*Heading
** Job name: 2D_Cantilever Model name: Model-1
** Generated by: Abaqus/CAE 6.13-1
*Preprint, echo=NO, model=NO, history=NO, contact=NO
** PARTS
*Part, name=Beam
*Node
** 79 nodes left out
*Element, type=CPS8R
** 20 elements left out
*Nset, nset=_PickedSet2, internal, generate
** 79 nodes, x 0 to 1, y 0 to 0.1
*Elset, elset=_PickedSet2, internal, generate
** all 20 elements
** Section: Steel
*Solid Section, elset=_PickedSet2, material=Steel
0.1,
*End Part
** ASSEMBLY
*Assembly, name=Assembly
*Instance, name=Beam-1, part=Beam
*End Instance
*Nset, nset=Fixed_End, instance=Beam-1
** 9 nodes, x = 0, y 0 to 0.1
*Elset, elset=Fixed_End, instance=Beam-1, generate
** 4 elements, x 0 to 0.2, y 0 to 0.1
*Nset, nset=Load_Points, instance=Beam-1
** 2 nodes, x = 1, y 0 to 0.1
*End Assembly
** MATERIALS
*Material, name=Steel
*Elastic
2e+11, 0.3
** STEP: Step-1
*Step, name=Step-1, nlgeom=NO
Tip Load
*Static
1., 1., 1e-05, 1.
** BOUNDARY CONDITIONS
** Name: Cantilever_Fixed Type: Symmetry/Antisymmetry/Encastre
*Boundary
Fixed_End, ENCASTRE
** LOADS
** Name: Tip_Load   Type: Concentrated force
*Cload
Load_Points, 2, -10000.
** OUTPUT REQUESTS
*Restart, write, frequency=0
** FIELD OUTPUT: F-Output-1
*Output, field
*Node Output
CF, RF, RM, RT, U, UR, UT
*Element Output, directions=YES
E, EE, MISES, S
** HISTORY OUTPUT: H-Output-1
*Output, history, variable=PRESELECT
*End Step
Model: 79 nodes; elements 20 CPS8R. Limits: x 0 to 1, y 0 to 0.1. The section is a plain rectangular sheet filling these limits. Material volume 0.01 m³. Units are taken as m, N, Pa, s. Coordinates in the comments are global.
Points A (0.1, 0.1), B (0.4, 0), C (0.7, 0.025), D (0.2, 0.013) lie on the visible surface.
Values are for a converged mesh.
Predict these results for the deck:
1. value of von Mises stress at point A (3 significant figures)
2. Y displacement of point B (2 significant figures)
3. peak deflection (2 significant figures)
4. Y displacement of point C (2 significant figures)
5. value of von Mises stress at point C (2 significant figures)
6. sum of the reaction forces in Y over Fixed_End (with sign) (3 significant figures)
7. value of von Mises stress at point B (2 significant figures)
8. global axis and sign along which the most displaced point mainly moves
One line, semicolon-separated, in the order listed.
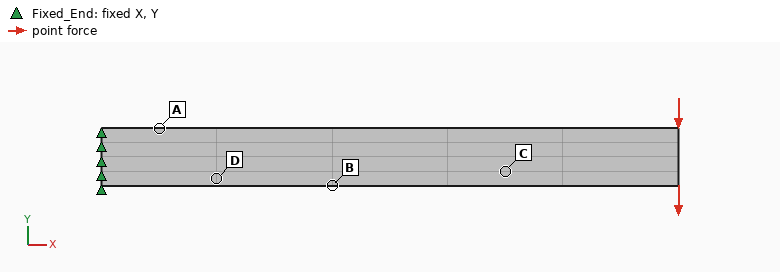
1.05e+08 Pa; -8.2e-04 m; 0.0039 m; -0.0022 m; 1.8e+07 Pa; 20000 N; 6.9e+07 Pa; -Y
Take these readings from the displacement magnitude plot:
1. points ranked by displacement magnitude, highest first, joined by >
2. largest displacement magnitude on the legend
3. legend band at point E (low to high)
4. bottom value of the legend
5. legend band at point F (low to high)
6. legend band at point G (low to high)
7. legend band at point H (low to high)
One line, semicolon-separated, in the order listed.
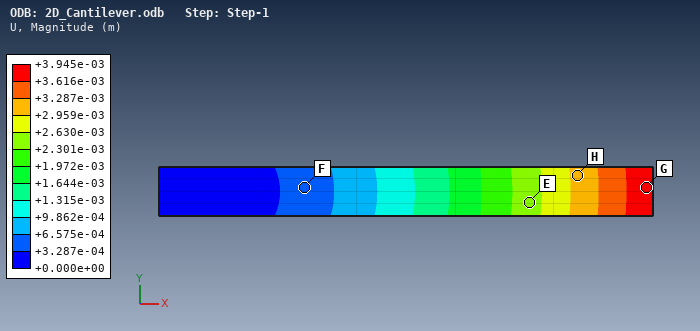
G > H > E > F; +3.945e-03 m; +2.301e-03 to +2.630e-03 m; +0.000e+00 m; +3.287e-04 to +6.575e-04 m; +3.616e-03 to +3.945e-03 m; +2.959e-03 to +3.287e-03 m
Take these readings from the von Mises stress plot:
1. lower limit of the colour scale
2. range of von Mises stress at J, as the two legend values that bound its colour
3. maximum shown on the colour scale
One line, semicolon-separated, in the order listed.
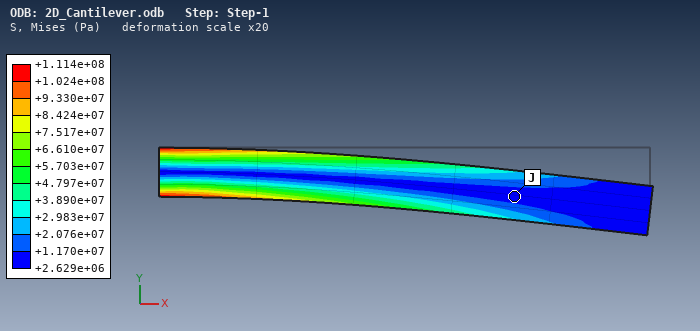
+2.629e+06 Pa; +2.629e+06 to +1.170e+07 Pa; +1.114e+08 Pa
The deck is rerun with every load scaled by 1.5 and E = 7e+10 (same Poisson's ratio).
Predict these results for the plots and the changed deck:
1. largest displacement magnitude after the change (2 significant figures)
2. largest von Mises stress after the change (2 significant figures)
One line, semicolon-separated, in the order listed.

0.017 m; 1.7e+08 Pa
